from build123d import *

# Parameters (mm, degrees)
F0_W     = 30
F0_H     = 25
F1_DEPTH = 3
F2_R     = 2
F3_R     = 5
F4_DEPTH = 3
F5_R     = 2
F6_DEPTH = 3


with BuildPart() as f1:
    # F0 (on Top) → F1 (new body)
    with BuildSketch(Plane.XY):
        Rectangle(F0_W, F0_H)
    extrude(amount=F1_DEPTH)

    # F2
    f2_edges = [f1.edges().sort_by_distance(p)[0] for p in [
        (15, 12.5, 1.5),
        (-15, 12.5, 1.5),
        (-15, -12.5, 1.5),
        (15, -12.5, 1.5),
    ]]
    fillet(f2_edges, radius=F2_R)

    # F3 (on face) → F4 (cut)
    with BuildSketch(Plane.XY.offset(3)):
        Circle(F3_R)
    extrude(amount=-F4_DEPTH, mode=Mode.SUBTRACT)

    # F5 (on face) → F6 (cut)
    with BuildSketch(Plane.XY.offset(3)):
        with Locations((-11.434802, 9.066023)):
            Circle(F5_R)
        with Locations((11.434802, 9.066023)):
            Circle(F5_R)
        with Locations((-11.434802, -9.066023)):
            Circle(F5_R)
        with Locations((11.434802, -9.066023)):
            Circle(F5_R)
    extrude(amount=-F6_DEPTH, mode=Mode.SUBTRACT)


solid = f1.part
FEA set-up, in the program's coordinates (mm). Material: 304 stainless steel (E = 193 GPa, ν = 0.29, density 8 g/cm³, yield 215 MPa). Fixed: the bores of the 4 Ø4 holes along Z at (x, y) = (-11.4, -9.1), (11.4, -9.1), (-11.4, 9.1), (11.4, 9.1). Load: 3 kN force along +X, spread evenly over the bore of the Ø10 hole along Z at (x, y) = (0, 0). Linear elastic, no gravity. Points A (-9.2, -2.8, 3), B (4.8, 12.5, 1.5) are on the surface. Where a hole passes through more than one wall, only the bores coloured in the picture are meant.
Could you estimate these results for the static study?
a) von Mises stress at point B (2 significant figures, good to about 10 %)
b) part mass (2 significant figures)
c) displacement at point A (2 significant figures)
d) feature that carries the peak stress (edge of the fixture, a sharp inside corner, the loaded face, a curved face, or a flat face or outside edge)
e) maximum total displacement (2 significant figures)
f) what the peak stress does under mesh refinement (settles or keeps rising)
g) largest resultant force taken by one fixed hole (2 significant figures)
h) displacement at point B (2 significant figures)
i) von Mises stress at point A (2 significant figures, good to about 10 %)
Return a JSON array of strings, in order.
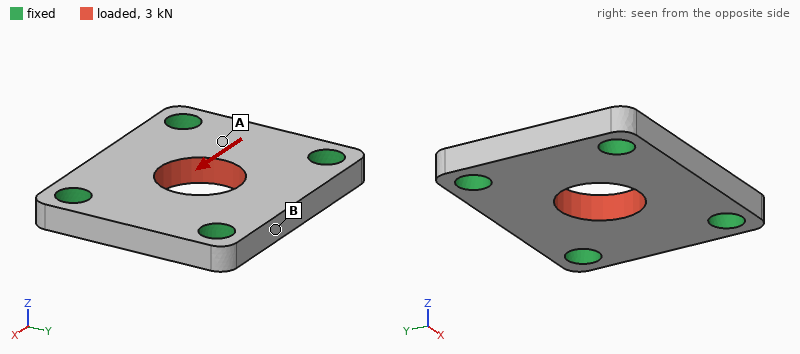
["6.8 MPa", "15 g", "1.3 µm", "edge of the fixture", "2.0 µm", "keeps rising", "800 N", "0.40 µm", "23 MPa"]
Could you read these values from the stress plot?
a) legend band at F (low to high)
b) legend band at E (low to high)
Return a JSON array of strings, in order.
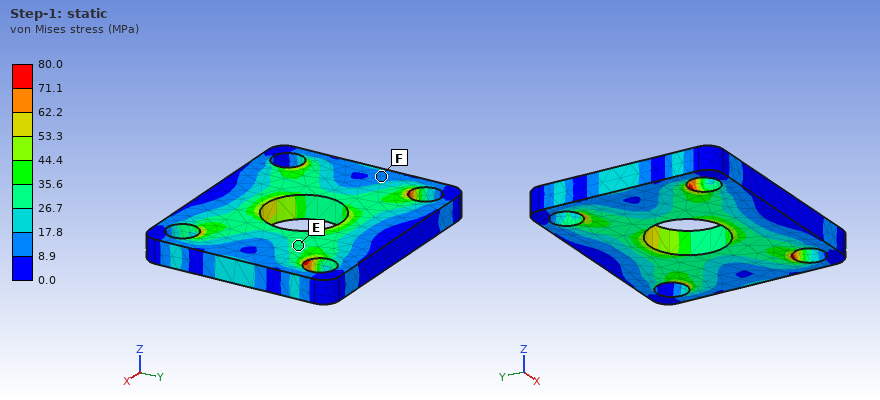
["8.9 to 17.8 MPa", "26.7 to 35.6 MPa"]
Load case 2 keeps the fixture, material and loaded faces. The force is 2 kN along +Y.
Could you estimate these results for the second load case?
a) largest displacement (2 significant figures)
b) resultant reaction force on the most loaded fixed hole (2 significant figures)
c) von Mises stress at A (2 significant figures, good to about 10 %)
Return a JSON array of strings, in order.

["2.1 µm", "560 N", "22 MPa"]
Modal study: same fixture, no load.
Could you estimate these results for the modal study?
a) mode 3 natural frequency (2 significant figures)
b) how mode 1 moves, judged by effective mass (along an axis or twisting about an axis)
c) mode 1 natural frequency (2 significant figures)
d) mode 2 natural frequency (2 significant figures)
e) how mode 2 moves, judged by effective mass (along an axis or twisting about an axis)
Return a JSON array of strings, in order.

["44 kHz", "along Z", "31 kHz", "36 kHz", "twisting about X"]
